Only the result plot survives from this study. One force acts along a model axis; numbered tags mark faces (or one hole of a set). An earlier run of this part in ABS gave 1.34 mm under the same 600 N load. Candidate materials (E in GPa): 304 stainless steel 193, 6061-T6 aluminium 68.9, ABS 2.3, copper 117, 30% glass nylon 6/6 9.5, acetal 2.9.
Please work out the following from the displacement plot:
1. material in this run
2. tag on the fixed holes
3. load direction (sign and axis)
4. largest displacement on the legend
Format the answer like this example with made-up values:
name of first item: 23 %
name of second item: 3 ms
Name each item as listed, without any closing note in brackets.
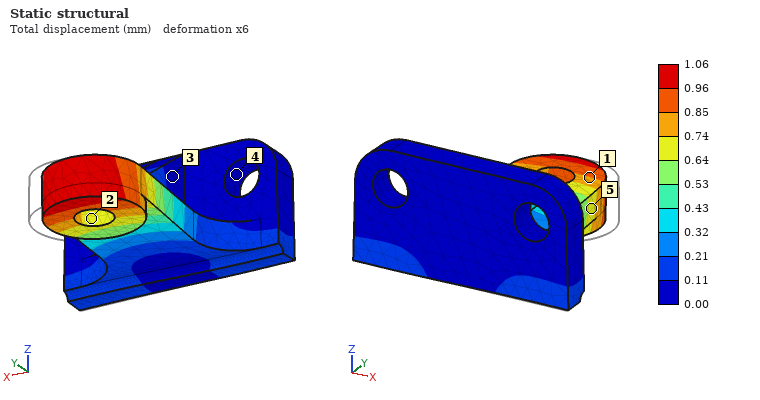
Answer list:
material in this run: acetal
tag on the fixed holes: 4
load direction: -X
largest displacement on the legend: 1.06 mm
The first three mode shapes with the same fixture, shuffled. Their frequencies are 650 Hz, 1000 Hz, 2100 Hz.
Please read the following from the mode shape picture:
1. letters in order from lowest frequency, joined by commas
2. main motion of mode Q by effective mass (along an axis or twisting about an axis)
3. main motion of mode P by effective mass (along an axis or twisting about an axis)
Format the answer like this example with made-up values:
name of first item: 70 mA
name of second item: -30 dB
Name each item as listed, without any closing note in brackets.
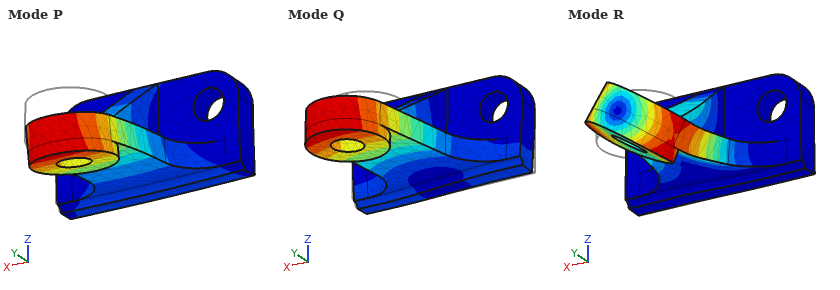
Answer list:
letters in order from lowest frequency, joined by commas: P, Q, R
main motion of mode Q by effective mass: along X
main motion of mode P by effective mass: along Z
